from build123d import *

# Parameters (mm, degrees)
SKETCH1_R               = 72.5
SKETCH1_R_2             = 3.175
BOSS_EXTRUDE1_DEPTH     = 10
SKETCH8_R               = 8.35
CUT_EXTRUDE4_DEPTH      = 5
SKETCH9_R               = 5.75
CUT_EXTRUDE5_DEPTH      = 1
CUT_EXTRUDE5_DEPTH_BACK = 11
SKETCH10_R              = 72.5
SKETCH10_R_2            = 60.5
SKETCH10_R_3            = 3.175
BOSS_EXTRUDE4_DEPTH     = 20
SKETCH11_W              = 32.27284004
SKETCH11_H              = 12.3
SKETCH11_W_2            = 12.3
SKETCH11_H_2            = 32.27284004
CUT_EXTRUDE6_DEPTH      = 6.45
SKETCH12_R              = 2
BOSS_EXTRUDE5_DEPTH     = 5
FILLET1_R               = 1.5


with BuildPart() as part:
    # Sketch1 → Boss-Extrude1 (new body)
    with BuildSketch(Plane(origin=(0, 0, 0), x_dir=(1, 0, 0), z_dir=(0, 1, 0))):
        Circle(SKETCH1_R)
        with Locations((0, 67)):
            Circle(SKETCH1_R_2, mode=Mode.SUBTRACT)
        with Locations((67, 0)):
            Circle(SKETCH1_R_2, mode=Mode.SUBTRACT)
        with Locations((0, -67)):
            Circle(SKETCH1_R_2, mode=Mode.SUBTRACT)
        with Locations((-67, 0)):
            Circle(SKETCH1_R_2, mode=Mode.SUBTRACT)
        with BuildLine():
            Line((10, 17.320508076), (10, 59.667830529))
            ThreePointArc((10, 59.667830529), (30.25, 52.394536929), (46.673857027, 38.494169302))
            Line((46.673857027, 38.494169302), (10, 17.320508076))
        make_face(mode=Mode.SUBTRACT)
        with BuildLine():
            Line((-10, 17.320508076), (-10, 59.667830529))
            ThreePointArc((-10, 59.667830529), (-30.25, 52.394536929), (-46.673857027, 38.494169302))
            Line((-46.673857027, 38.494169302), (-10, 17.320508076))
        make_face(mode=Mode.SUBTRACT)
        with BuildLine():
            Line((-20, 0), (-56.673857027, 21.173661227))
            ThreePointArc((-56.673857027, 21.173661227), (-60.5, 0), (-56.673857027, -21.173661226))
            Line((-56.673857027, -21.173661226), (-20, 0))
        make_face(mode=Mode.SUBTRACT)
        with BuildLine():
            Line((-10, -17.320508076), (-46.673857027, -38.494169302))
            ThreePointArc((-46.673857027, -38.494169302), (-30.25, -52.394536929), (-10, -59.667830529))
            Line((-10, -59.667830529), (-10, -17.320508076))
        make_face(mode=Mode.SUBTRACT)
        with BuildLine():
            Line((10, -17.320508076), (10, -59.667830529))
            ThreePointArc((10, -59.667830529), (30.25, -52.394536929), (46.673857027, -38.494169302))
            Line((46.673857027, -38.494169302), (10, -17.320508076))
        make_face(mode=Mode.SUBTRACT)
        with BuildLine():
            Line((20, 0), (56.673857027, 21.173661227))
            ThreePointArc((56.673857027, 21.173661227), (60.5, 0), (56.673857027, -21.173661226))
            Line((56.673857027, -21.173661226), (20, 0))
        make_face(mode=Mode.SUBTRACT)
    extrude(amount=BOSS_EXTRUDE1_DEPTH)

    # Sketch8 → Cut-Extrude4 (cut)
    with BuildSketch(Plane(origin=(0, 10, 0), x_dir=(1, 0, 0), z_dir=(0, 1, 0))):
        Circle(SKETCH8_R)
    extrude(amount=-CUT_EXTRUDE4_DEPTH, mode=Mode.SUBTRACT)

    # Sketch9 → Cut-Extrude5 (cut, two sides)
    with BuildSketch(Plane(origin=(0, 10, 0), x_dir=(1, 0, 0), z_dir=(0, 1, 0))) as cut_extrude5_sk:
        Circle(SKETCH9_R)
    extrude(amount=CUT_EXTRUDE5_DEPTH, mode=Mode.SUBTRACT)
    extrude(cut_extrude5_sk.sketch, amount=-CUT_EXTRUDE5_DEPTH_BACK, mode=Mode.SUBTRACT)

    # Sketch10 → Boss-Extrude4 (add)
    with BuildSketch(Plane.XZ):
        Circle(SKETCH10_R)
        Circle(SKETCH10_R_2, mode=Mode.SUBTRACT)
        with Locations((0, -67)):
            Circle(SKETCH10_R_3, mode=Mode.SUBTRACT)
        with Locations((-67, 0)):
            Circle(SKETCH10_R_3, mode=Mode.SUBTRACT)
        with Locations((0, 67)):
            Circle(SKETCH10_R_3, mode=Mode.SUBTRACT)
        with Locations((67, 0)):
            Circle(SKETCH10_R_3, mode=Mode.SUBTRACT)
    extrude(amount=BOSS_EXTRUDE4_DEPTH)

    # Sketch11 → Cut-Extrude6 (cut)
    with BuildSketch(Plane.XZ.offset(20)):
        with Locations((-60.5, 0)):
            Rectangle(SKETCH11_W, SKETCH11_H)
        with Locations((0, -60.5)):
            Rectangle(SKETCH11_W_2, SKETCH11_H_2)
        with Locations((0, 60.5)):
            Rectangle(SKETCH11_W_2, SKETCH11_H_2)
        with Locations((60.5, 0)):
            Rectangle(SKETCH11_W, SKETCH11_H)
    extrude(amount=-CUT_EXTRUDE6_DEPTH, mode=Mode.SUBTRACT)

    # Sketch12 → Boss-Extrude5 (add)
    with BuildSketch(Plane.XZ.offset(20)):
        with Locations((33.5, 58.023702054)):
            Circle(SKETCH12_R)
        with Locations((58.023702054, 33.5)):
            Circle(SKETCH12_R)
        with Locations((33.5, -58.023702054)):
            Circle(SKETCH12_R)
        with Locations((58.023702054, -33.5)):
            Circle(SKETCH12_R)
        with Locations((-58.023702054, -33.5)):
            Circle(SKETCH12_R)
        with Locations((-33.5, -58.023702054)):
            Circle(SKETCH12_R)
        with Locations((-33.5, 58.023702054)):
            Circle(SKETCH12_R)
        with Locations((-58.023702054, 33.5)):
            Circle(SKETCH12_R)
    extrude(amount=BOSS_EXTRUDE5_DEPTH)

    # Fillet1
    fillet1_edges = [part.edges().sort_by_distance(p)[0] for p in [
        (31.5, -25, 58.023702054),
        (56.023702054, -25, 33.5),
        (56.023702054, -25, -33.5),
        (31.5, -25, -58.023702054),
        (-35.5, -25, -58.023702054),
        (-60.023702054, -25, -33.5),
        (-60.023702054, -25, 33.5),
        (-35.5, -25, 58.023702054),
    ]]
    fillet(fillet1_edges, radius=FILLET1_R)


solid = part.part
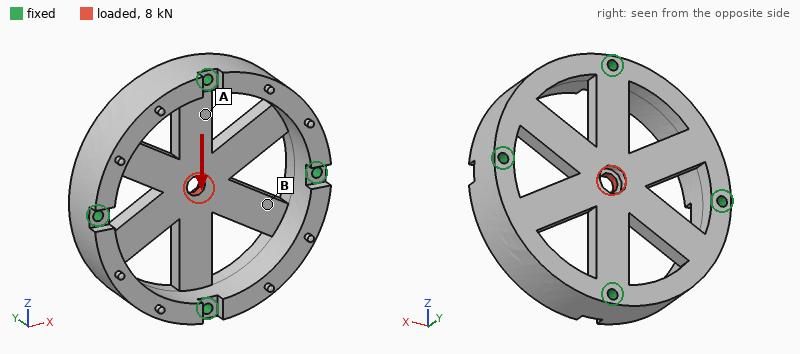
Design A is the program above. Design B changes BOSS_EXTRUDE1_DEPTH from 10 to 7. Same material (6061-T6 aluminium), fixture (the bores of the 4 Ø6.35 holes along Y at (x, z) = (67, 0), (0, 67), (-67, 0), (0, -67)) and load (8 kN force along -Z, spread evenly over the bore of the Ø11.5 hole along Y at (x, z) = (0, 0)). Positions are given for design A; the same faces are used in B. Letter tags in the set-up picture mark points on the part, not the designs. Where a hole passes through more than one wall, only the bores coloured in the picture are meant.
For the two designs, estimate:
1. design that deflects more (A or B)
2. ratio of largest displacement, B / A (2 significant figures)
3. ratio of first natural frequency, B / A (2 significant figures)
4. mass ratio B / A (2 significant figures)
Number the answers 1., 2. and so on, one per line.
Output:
1. B
2. 1.2
3. 0.77
4. 0.84
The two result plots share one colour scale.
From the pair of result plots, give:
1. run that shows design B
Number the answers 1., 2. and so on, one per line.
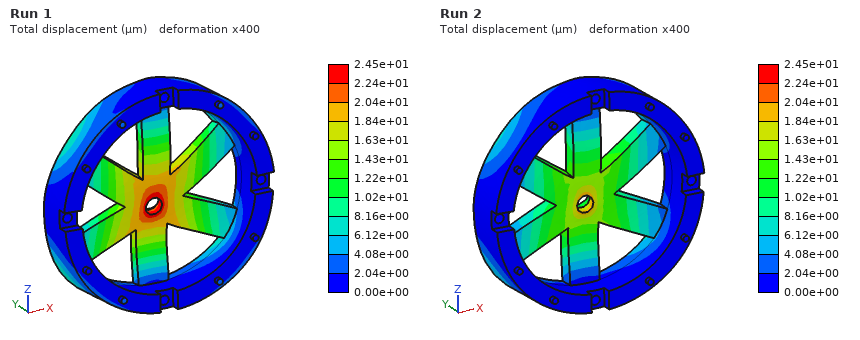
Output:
1. Run 1
